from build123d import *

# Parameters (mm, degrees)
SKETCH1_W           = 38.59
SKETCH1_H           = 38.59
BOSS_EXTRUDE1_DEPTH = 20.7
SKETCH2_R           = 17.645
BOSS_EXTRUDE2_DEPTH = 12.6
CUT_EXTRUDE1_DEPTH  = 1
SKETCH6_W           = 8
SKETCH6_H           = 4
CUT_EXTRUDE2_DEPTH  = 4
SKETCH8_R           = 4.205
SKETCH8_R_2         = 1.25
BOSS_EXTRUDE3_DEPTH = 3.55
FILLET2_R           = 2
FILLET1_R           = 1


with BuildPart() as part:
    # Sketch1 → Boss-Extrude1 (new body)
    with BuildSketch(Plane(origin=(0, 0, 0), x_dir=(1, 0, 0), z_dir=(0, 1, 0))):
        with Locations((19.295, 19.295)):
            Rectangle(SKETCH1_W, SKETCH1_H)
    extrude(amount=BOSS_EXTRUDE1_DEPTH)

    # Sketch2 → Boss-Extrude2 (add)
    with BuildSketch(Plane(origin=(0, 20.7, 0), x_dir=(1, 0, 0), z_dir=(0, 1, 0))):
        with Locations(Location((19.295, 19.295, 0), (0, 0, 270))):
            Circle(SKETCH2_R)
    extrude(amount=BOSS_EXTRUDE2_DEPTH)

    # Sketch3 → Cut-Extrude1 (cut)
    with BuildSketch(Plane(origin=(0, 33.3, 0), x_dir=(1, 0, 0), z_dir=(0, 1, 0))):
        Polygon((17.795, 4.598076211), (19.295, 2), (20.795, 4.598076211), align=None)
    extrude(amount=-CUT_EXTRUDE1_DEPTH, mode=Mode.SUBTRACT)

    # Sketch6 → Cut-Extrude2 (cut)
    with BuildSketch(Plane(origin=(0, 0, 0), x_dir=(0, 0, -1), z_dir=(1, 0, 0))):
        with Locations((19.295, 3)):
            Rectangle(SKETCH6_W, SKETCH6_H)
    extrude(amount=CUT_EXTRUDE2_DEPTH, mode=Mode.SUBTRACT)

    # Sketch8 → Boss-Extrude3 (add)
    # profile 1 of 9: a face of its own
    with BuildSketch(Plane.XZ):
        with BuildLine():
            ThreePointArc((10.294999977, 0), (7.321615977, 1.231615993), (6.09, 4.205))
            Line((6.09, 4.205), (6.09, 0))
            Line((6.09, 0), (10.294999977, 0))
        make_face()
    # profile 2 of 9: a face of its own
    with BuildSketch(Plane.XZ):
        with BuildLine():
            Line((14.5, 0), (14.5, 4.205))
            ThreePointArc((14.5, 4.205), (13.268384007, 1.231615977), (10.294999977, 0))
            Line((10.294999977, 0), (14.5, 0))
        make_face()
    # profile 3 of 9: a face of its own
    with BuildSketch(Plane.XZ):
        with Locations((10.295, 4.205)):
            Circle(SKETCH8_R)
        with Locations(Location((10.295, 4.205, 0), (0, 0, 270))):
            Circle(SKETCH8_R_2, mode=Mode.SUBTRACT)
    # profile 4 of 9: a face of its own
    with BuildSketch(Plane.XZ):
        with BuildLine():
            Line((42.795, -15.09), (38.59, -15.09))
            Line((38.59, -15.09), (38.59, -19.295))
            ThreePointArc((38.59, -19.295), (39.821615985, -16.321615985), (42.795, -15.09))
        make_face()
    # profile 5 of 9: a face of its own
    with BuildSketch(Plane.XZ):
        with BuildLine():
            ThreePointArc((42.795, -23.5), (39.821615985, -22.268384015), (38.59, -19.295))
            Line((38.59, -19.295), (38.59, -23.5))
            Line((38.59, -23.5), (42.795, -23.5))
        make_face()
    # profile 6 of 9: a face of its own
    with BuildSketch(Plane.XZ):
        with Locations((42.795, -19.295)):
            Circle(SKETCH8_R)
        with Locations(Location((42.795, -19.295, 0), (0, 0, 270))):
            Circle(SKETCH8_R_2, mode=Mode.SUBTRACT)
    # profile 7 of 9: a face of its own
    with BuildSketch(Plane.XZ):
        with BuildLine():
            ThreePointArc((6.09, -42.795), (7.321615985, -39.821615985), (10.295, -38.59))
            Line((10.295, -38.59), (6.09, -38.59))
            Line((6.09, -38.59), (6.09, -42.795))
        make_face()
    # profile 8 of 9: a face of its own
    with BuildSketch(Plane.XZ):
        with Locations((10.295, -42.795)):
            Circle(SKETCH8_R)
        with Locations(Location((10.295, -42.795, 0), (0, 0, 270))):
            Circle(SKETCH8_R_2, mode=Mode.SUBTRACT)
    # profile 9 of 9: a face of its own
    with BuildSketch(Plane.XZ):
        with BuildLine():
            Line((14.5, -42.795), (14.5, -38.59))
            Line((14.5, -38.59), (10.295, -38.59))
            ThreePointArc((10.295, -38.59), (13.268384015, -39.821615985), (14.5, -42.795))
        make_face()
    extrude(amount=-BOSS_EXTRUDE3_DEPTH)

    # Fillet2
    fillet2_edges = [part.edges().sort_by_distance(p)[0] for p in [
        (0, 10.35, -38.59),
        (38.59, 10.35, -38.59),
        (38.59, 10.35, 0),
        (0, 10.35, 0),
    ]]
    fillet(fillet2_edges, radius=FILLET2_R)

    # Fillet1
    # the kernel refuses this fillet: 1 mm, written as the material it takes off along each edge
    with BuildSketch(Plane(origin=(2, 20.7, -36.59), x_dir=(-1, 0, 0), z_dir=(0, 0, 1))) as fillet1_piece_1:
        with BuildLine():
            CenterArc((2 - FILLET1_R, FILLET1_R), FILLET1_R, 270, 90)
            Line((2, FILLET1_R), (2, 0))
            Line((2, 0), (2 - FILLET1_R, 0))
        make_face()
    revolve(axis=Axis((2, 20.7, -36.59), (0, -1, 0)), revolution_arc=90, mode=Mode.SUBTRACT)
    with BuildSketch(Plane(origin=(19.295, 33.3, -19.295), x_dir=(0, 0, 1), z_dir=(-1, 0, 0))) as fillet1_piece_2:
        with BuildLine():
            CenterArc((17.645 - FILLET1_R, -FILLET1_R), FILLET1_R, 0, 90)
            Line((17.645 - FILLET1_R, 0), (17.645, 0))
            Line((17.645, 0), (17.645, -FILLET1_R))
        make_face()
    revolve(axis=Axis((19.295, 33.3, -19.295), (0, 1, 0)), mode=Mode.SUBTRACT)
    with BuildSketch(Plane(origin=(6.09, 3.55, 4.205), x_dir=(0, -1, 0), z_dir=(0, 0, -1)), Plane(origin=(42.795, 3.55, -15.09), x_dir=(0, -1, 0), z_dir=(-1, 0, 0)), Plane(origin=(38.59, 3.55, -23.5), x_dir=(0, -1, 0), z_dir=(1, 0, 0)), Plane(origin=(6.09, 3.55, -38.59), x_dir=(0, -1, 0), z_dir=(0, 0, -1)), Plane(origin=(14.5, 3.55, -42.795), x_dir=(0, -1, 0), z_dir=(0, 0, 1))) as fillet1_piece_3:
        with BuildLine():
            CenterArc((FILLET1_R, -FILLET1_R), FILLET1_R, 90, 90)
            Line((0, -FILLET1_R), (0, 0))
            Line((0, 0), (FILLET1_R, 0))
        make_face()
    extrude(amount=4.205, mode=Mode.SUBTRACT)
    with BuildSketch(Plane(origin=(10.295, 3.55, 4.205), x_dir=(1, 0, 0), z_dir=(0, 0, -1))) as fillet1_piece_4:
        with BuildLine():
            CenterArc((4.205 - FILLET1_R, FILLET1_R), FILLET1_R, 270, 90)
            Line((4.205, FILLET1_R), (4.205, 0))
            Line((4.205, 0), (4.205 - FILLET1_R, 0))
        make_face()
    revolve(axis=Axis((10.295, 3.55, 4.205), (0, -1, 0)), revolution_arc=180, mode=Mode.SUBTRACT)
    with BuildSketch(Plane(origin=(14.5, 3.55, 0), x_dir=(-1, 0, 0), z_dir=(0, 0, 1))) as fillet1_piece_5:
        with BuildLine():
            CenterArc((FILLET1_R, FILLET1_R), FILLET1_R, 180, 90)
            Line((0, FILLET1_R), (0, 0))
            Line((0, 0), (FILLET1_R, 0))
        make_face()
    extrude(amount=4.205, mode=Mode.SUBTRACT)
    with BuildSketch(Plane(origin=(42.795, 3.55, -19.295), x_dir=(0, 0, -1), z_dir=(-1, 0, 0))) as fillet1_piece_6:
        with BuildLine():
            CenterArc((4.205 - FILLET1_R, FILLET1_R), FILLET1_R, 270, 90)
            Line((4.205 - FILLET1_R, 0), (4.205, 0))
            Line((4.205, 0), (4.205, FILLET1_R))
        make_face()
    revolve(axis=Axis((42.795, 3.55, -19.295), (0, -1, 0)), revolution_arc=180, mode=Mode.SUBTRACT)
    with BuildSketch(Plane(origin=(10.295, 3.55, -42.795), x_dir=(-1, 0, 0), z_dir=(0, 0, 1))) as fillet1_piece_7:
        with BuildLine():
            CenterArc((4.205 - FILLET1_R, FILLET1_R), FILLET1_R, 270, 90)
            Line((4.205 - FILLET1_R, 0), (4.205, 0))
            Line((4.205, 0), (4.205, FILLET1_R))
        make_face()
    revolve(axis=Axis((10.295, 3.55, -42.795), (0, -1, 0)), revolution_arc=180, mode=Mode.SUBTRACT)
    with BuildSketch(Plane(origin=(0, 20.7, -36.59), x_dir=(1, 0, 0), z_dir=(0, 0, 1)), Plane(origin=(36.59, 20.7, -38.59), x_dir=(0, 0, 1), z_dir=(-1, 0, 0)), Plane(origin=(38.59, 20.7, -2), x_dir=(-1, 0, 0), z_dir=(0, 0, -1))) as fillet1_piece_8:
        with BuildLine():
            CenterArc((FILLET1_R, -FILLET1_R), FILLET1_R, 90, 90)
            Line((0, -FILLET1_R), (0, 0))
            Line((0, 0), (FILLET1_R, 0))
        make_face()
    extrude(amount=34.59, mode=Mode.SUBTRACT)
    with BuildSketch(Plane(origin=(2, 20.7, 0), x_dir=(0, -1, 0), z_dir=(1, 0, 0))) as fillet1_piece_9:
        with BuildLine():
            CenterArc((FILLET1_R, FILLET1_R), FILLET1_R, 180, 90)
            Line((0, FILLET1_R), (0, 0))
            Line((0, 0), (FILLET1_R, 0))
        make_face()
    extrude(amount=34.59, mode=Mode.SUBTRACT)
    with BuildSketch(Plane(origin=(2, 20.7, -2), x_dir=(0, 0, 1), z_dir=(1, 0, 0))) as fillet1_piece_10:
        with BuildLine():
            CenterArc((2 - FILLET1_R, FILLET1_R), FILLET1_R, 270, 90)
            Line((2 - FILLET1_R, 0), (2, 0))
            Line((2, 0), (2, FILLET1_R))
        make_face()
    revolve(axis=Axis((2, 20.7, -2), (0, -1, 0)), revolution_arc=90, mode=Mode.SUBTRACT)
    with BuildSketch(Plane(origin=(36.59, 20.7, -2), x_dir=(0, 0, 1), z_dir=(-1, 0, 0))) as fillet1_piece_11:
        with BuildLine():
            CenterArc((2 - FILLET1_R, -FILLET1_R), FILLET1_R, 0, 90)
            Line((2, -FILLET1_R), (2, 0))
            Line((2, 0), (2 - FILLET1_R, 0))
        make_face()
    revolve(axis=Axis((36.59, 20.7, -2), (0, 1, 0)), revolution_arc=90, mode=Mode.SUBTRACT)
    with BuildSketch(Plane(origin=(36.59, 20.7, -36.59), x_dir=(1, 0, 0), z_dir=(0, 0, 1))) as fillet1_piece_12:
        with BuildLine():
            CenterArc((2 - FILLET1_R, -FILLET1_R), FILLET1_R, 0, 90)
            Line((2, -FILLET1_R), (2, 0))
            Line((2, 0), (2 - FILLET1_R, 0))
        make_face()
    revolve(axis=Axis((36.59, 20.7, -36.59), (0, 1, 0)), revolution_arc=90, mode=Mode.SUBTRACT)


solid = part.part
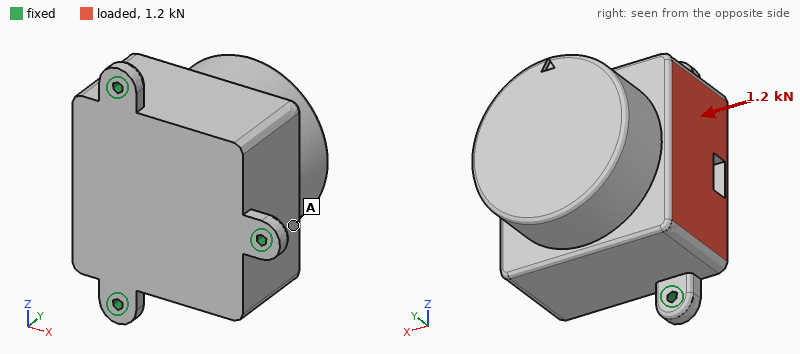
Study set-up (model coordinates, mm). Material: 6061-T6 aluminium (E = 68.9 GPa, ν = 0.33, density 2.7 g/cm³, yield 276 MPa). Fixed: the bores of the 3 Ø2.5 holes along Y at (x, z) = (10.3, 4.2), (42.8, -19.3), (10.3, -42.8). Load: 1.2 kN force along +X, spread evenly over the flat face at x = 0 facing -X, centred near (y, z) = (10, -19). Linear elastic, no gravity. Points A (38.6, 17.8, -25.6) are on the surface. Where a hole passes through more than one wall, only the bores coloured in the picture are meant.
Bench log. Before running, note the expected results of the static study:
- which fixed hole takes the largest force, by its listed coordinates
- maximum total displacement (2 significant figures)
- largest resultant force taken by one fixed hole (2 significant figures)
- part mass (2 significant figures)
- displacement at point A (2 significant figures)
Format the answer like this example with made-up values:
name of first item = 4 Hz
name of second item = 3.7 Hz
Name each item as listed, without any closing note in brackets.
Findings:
which fixed hole takes the largest force, by its listed coordinates = (42.8, -19.3)
maximum total displacement = 11 µm
largest resultant force taken by one fixed hole = 760 N
part mass = 120 g
displacement at point A = 7.5 µm
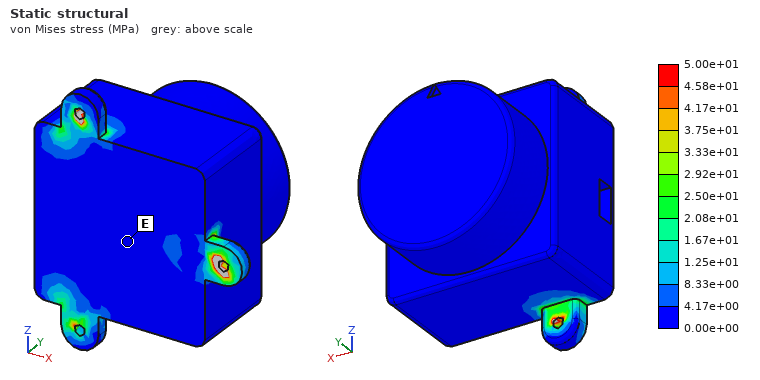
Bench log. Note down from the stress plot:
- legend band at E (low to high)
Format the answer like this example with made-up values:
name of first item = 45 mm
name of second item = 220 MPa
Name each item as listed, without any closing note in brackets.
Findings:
legend band at E = 0.00e+00 to 4.17e+00 MPa
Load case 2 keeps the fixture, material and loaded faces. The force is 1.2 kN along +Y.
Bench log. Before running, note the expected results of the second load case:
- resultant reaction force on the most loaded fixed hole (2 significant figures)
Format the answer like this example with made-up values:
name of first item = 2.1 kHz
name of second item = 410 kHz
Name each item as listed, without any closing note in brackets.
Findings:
resultant reaction force on the most loaded fixed hole = 880 N
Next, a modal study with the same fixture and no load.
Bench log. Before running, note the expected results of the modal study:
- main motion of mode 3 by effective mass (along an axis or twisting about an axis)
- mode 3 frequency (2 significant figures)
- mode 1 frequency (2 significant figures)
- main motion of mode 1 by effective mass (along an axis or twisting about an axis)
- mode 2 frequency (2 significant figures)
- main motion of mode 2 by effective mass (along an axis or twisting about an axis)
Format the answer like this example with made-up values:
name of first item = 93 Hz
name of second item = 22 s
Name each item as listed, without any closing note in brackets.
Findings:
main motion of mode 3 by effective mass = along Y
mode 3 frequency = 6400 Hz
mode 1 frequency = 4500 Hz
main motion of mode 1 by effective mass = along X
mode 2 frequency = 5400 Hz
main motion of mode 2 by effective mass = along Z
